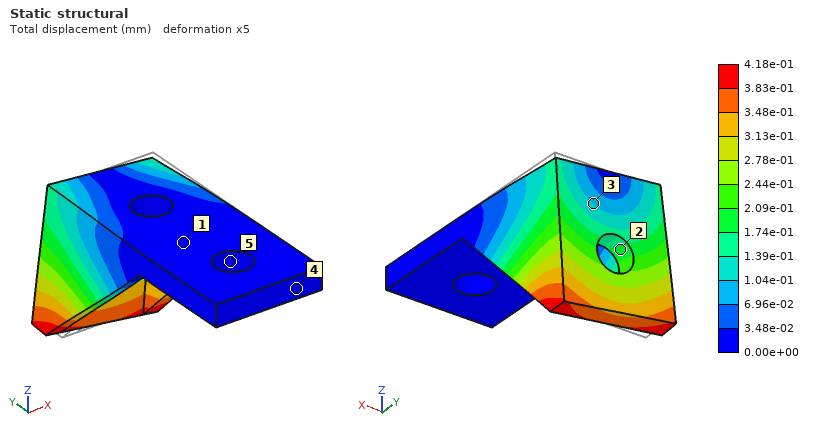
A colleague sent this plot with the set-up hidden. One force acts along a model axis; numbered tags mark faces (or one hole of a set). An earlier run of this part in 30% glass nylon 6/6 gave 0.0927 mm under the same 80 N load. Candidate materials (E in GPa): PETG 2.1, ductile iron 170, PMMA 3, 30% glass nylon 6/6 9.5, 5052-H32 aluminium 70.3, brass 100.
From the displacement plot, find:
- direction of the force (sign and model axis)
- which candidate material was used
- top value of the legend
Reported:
-X
PETG
4.18e-01 mm
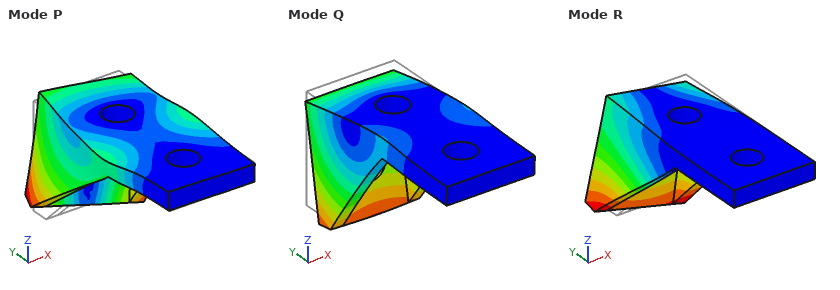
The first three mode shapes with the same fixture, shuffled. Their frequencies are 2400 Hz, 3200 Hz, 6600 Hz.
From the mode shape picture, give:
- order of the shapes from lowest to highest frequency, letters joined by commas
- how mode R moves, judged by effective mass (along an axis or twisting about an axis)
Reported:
R, Q, P
along X
